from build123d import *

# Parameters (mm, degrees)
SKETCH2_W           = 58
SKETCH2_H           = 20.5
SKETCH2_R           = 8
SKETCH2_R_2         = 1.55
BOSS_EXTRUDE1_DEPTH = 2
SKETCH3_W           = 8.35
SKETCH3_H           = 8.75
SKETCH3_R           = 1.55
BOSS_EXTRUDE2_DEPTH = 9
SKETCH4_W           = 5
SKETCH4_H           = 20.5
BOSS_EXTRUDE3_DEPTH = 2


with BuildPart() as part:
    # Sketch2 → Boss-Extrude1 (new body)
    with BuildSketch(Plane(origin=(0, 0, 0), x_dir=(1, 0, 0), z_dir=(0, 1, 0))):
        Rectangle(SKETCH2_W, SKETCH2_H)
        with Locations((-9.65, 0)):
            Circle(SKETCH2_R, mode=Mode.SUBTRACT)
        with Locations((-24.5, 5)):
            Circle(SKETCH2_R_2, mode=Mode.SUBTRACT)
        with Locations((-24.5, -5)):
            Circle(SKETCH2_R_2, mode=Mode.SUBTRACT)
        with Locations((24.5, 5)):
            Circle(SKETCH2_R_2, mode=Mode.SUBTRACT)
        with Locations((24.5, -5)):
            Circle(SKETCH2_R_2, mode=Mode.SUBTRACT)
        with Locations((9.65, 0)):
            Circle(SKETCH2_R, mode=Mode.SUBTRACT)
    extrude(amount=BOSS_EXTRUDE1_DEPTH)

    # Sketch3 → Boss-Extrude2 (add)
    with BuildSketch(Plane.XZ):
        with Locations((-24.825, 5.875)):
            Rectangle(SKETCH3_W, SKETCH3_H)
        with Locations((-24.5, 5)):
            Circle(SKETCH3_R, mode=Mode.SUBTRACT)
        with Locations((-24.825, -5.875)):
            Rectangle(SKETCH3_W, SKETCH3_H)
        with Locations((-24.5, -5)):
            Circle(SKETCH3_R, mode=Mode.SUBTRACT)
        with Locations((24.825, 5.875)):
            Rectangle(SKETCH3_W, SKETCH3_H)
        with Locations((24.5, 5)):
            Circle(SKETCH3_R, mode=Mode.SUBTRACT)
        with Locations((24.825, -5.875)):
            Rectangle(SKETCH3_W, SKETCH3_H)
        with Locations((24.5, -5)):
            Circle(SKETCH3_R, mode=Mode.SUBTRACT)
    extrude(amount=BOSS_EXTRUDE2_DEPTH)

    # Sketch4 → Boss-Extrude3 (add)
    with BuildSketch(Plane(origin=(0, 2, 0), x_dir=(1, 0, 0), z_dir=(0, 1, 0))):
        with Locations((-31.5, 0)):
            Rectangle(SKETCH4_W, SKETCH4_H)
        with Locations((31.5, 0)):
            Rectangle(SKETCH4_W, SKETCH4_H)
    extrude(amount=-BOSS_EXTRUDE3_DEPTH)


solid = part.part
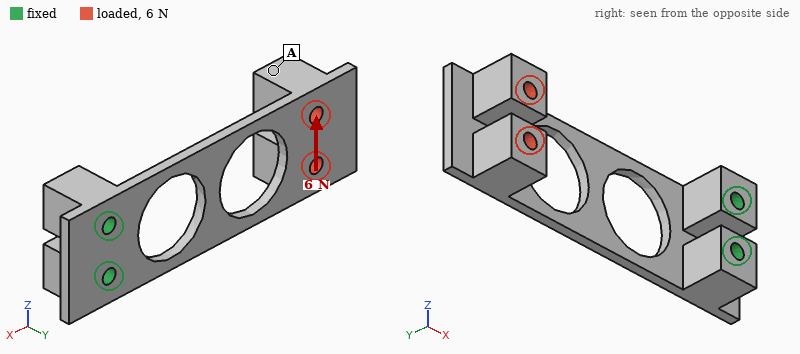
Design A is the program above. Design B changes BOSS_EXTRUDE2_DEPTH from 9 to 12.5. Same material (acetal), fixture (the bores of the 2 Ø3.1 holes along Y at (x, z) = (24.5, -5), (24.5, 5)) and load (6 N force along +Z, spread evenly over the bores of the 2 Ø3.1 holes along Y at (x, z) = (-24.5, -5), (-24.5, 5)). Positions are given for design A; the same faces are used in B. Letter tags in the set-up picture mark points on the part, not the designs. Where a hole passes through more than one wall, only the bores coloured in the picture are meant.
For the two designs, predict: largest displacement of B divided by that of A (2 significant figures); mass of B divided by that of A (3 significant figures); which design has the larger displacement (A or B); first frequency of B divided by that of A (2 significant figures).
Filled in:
1.5
1.21
B
0.89
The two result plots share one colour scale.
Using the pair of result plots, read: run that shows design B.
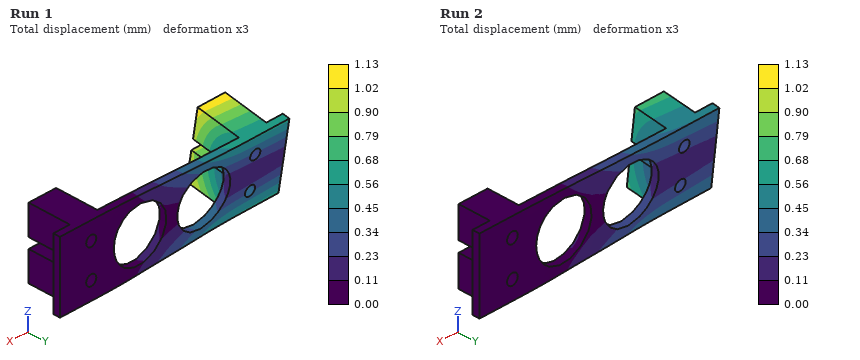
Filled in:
Run 1
